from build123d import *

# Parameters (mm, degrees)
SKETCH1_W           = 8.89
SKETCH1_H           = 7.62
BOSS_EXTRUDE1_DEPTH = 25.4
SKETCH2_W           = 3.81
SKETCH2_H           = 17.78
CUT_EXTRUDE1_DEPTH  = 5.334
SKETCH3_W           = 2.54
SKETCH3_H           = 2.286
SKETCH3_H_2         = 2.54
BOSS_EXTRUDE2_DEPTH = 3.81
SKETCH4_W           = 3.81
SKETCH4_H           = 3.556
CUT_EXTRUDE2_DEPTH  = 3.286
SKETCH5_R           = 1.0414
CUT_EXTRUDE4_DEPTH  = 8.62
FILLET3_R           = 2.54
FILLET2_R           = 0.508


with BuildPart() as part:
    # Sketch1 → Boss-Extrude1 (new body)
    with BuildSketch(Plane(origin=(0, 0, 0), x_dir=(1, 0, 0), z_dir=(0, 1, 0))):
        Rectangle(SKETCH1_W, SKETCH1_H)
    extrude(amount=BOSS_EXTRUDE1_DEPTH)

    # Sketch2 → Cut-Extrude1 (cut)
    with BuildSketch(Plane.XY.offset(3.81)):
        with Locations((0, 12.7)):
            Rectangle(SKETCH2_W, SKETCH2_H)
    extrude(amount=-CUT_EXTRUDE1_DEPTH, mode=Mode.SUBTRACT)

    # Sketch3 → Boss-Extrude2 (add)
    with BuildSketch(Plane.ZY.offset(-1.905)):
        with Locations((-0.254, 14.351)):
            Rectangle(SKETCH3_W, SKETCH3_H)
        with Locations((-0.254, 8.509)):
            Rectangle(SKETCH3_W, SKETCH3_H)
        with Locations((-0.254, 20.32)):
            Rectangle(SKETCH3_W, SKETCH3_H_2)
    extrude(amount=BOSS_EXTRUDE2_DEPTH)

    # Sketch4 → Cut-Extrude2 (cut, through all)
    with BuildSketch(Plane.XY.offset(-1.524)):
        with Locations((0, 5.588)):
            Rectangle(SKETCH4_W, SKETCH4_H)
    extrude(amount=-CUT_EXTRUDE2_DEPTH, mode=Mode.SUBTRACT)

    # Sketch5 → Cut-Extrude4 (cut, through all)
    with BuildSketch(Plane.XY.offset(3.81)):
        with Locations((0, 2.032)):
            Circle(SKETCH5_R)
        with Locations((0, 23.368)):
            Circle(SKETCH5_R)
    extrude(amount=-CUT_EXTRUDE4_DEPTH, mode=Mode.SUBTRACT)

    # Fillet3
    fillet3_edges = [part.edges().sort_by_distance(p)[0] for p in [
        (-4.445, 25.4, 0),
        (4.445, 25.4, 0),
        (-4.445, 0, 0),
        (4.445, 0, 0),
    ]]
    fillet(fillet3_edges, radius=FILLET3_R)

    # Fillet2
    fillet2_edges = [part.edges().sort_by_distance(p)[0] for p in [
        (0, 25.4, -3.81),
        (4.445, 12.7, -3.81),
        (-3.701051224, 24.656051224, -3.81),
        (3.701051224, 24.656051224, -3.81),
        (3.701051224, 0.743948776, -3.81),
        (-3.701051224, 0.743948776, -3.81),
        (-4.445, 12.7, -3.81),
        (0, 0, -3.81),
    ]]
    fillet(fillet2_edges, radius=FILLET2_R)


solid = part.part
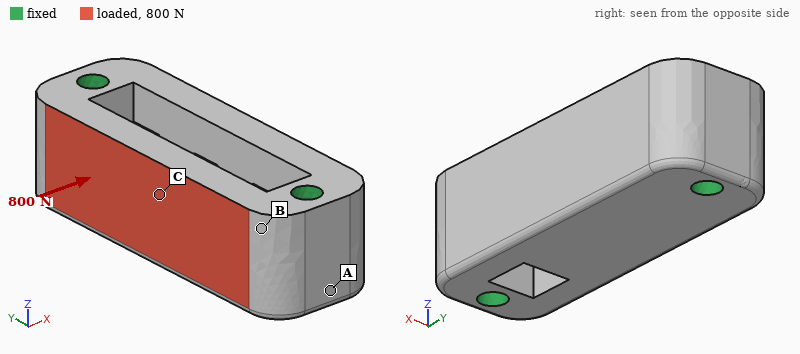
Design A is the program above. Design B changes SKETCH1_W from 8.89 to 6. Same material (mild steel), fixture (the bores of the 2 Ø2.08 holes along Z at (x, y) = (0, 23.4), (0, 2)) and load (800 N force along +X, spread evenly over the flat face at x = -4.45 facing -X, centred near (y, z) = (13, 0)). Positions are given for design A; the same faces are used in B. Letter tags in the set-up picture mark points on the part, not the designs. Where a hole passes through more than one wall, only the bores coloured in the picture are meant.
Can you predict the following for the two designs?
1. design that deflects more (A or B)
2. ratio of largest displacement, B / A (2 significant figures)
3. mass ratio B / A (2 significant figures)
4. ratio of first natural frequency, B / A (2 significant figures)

B
3.7
0.57
0.76
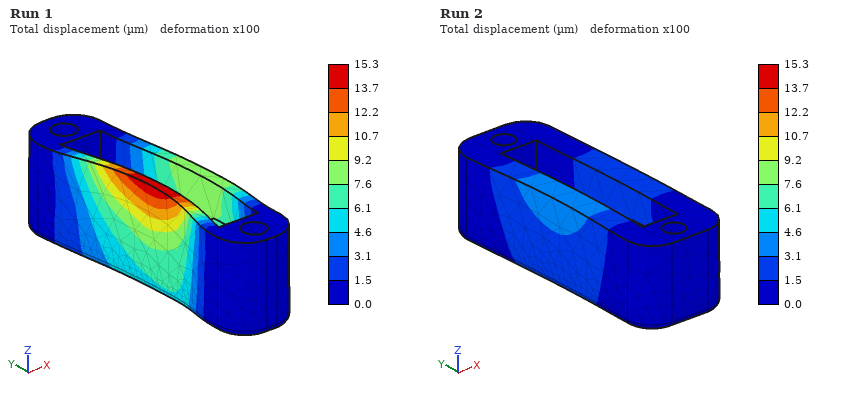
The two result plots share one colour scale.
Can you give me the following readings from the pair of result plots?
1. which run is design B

Run 1
